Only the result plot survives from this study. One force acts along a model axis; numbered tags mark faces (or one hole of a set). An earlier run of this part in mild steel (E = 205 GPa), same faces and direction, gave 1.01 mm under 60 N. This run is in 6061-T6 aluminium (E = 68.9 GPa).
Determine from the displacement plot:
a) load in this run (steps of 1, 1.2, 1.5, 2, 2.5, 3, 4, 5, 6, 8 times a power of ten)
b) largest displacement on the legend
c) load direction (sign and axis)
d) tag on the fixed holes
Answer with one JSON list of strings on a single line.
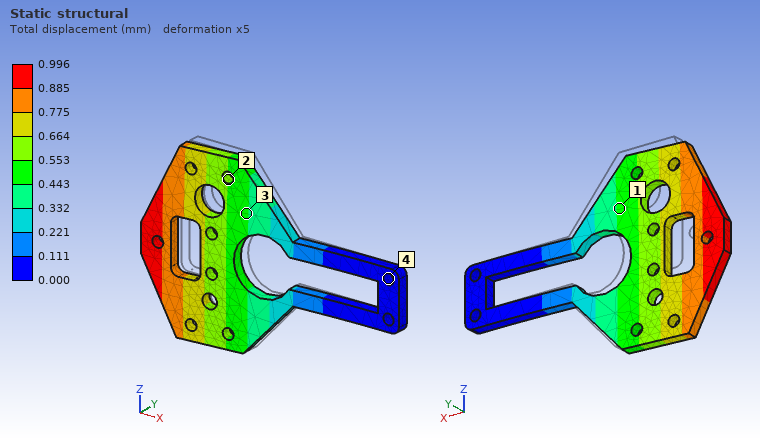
["20 N", "0.996 mm", "-Y", "4"]
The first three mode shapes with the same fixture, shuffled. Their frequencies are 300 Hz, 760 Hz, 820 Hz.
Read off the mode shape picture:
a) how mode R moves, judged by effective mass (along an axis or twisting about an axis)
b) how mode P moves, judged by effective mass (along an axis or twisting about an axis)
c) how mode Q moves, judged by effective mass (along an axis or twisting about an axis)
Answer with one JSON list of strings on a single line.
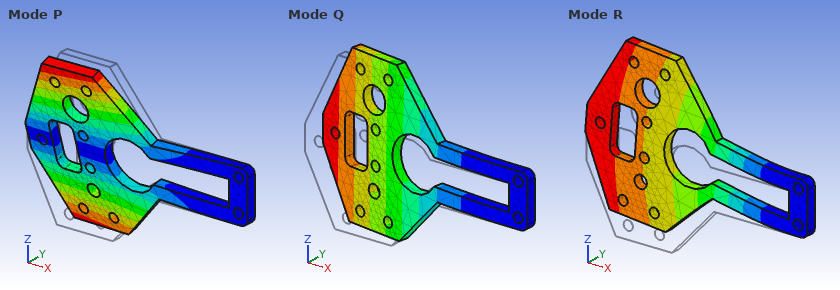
["along Z", "twisting about X", "along Y"]
